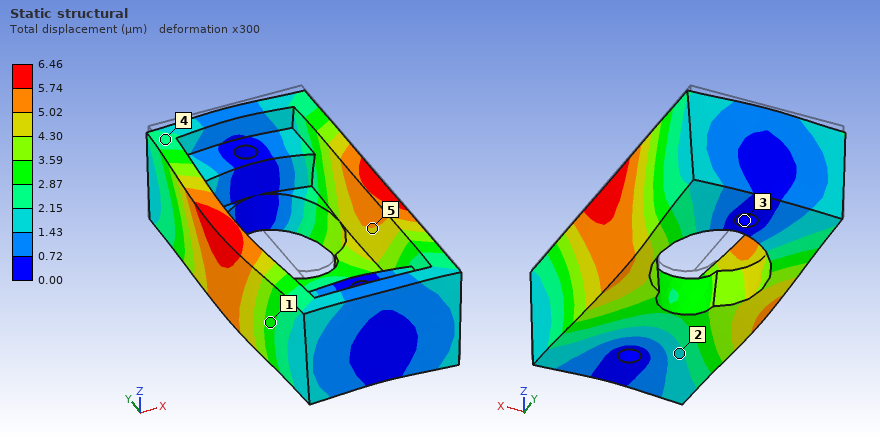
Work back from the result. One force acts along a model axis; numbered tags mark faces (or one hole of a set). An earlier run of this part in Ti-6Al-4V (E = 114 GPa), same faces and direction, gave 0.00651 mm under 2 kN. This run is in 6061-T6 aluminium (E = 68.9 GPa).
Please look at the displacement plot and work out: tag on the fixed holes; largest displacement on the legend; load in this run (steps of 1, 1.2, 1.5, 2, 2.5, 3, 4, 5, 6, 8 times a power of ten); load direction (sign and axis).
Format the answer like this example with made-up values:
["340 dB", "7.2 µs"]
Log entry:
["3", "6.46 µm", "1.2 kN", "-Z"]
